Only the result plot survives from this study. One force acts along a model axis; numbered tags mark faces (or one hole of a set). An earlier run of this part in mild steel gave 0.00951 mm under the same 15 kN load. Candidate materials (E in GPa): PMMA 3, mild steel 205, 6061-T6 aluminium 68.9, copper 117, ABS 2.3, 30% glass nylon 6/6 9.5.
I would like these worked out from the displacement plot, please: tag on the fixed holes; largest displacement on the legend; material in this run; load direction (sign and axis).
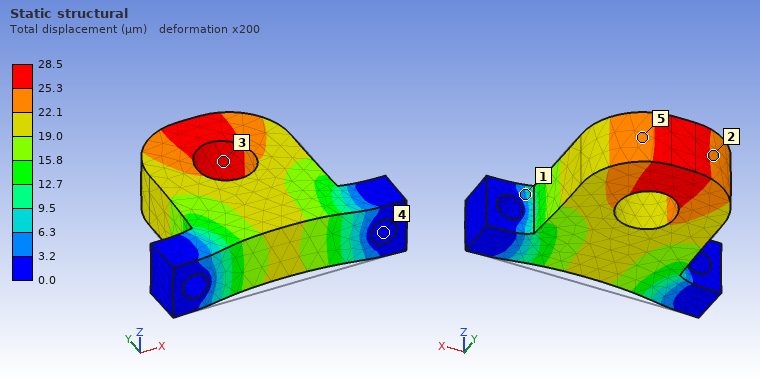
4
28.5 µm
6061-T6 aluminium
+Y
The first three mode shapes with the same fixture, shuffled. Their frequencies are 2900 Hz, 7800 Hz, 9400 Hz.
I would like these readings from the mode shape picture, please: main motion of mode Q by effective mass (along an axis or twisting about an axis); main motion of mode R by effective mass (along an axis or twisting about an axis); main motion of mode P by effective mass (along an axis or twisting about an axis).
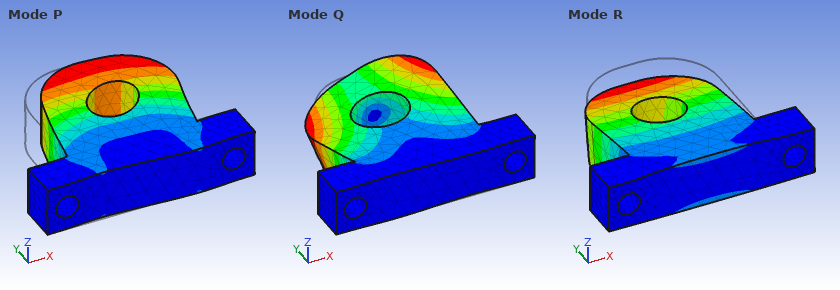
twisting about Y
along Z
along X
